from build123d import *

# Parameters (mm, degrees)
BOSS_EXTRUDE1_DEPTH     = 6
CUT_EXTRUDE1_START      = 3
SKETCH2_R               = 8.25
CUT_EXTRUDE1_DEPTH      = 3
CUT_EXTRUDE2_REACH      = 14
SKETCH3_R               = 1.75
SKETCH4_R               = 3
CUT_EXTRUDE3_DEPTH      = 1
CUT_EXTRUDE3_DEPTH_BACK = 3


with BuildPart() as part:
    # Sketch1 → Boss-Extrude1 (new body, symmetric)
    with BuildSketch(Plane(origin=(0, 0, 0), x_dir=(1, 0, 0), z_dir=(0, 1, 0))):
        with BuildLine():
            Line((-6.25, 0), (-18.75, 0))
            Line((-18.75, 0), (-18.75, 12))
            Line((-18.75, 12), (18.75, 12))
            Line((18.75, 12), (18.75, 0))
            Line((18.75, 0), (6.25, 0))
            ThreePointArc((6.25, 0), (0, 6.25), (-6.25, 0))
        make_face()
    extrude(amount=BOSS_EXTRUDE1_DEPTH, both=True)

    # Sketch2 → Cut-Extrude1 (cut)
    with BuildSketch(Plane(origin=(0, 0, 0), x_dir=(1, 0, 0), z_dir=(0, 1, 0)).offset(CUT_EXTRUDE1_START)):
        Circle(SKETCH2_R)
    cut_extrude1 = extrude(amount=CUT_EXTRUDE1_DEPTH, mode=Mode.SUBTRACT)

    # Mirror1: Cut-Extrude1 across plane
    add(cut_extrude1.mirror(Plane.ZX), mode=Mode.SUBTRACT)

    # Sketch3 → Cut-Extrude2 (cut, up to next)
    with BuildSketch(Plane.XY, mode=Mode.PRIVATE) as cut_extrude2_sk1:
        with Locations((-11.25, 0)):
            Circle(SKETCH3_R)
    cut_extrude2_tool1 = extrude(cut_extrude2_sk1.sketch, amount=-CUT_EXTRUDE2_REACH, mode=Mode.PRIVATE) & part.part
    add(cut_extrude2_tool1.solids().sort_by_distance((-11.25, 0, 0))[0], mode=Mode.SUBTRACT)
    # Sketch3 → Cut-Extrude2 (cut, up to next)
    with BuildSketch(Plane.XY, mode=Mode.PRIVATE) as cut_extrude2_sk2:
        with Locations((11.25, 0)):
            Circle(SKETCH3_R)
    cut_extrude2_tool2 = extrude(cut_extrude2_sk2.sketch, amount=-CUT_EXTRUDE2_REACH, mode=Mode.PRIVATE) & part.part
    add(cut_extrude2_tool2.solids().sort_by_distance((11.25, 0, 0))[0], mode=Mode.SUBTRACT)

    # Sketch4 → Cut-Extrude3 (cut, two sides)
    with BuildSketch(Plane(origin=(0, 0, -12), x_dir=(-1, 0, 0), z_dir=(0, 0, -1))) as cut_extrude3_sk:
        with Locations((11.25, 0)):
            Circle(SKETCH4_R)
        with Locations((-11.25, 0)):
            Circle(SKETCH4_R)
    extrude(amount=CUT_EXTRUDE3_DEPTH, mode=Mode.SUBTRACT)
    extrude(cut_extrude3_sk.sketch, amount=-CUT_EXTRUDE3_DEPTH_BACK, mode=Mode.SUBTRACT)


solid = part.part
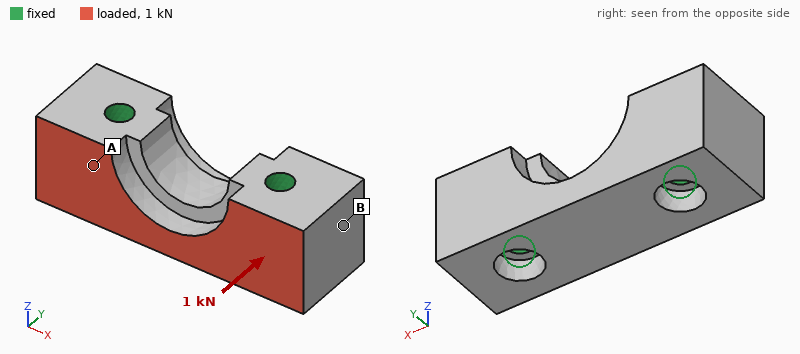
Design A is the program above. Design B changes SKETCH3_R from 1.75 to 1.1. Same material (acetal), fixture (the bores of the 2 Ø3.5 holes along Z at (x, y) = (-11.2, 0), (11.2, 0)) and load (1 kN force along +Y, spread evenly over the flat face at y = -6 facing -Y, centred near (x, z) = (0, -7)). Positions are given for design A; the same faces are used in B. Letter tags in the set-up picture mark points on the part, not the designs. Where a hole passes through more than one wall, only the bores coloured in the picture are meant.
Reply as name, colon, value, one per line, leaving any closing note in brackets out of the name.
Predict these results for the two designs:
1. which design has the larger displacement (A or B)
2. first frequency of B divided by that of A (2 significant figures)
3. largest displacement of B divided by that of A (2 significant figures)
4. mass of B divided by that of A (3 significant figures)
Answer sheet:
which design has the larger displacement: B
first frequency of B divided by that of A: 0.78
largest displacement of B divided by that of A: 1.2
mass of B divided by that of A: 1.03
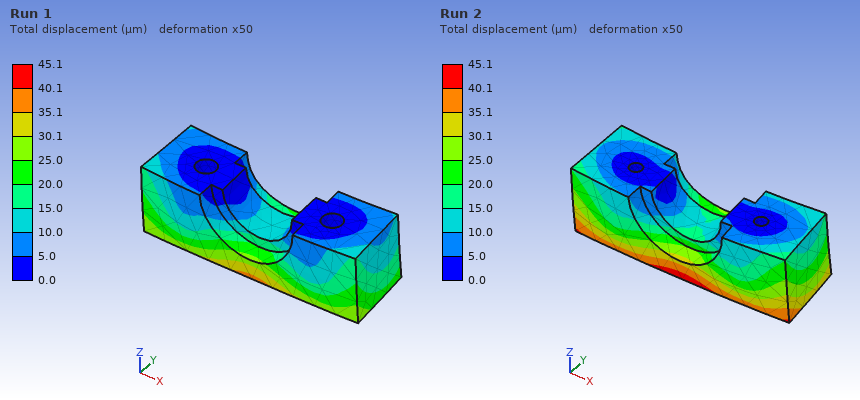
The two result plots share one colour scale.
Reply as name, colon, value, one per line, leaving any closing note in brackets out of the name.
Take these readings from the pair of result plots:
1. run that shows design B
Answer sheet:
run that shows design B: Run 2
